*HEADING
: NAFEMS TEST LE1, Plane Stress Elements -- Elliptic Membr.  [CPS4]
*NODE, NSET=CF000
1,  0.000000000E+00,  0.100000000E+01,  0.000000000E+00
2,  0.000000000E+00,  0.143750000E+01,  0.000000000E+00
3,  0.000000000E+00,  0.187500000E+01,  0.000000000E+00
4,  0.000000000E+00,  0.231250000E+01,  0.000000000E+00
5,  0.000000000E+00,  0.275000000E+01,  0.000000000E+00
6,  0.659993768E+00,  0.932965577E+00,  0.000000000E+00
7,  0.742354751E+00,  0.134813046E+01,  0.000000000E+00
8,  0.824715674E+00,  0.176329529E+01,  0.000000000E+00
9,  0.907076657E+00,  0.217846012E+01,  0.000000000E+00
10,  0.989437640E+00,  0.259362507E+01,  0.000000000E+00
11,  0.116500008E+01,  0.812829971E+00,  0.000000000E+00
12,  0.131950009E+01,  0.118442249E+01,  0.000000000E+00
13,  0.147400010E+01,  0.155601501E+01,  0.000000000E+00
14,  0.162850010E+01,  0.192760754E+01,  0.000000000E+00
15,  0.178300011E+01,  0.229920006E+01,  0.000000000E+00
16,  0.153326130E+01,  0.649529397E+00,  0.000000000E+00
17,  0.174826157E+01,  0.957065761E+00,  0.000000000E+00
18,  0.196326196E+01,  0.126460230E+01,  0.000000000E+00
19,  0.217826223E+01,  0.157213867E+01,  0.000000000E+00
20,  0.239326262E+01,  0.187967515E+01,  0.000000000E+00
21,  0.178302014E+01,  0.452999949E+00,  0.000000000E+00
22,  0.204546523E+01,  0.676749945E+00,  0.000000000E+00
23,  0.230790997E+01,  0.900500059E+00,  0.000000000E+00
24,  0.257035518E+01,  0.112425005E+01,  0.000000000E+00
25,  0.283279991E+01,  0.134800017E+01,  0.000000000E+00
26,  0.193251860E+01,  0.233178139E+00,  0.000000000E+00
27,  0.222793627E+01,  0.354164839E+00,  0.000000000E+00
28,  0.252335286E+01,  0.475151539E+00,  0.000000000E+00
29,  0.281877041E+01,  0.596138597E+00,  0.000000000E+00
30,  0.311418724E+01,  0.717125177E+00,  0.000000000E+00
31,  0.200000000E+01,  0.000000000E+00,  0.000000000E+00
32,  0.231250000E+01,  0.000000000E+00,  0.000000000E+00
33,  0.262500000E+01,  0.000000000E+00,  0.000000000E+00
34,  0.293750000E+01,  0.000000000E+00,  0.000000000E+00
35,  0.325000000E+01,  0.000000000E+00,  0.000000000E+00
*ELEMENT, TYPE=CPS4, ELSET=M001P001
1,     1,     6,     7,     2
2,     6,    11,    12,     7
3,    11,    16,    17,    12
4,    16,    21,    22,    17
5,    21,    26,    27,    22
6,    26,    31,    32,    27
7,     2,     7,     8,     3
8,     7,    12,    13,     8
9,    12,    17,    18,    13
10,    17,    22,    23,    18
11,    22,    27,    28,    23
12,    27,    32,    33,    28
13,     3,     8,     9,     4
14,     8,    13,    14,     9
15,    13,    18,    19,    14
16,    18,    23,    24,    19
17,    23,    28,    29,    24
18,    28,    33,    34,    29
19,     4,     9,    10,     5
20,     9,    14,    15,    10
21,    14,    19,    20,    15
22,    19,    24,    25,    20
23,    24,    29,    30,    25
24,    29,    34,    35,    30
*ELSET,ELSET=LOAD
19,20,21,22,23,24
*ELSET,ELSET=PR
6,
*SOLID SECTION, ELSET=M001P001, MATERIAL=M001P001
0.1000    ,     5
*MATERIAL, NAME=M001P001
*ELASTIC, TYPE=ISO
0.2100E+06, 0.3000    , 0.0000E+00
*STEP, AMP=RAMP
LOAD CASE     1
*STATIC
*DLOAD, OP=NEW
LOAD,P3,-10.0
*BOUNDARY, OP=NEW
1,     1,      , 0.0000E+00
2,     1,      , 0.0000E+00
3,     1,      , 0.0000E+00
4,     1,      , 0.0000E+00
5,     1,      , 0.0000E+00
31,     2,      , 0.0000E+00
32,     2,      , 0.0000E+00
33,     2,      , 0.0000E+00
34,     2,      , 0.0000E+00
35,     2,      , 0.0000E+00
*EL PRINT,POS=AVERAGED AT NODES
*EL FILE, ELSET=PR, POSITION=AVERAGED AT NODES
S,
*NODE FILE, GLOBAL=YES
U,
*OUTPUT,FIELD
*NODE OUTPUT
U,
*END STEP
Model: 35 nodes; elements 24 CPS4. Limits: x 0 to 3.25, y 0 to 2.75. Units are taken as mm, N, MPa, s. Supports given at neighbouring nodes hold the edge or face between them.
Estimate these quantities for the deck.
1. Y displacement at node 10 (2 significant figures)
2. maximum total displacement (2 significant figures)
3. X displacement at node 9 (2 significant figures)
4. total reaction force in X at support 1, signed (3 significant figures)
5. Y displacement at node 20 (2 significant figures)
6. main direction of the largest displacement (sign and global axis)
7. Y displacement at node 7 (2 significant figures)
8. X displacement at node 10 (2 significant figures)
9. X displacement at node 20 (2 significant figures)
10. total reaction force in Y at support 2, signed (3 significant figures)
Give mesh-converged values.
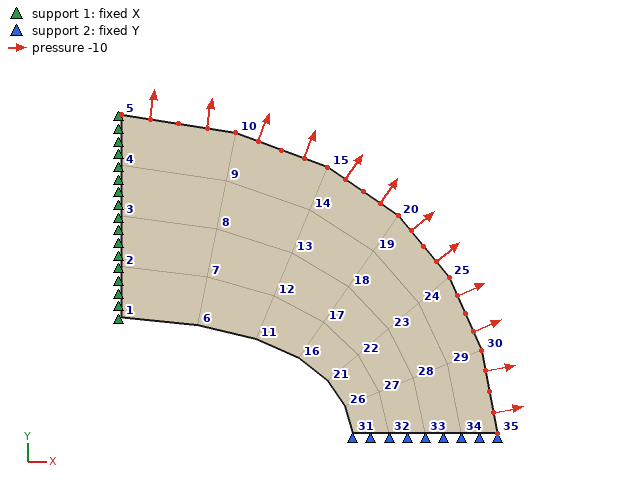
4.8e-04 mm
5.5e-04 mm
9.0e-05 mm
-2.75 N
1.7e-04 mm
+Y
5.0e-04 mm
1.3e-04 mm
1.5e-04 mm
-3.25 N
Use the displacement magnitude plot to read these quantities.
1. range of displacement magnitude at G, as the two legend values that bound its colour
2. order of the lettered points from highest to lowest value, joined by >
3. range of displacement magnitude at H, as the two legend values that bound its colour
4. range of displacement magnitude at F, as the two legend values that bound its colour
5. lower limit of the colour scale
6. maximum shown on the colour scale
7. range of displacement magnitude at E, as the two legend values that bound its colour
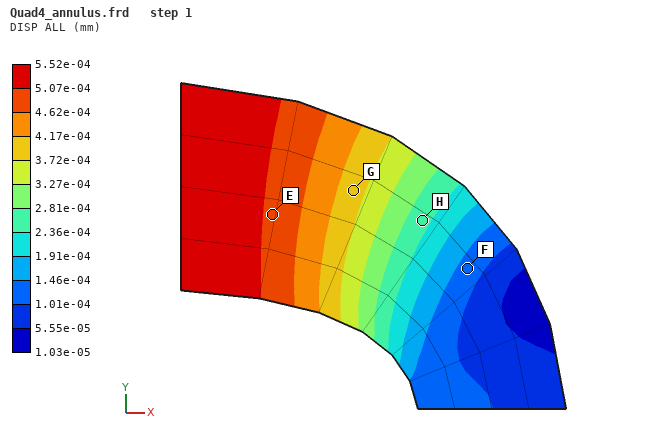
3.72e-04 to 4.17e-04 mm
E > G > H > F
2.36e-04 to 2.81e-04 mm
1.01e-04 to 1.46e-04 mm
1.03e-05 mm
5.52e-04 mm
4.62e-04 to 5.07e-04 mm
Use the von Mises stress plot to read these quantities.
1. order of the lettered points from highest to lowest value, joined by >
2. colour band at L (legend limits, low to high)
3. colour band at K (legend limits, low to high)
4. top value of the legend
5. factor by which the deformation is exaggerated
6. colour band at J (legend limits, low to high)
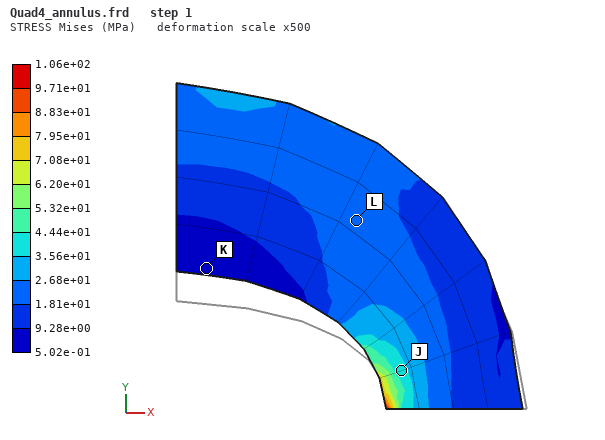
J > L > K
1.81e+01 to 2.68e+01 MPa
5.02e-01 to 9.28e+00 MPa
1.06e+02 MPa
500
3.56e+01 to 4.44e+01 MPa
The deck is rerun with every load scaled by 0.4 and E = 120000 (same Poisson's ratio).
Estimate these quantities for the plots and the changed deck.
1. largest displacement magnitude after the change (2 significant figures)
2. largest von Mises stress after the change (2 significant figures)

3.9e-04 mm
42 MPa
